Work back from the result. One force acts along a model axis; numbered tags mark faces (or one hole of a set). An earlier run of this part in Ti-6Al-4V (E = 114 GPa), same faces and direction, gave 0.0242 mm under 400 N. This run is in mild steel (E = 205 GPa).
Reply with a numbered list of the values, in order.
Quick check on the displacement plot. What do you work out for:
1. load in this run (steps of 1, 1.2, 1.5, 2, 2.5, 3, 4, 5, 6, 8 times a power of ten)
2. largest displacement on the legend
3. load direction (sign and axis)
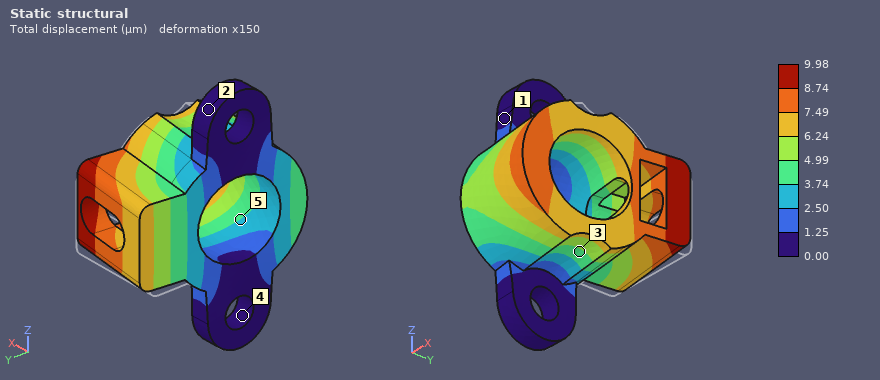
1. 300 N
2. 9.98 µm
3. -Y
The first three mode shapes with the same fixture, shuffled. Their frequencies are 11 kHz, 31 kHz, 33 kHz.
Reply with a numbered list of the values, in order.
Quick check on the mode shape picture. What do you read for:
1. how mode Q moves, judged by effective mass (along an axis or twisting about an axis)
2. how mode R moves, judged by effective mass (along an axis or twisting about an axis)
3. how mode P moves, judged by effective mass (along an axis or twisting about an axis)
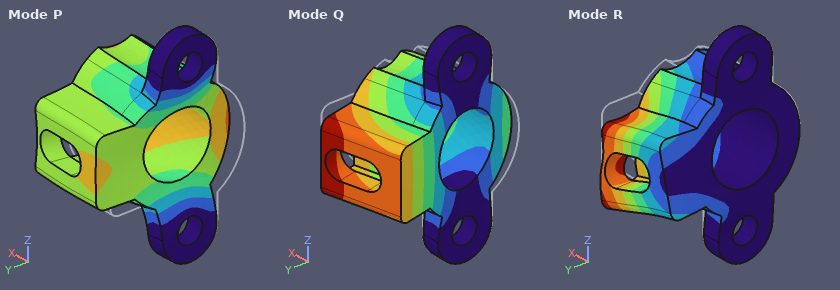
1. along Y
2. along Z
3. along X
